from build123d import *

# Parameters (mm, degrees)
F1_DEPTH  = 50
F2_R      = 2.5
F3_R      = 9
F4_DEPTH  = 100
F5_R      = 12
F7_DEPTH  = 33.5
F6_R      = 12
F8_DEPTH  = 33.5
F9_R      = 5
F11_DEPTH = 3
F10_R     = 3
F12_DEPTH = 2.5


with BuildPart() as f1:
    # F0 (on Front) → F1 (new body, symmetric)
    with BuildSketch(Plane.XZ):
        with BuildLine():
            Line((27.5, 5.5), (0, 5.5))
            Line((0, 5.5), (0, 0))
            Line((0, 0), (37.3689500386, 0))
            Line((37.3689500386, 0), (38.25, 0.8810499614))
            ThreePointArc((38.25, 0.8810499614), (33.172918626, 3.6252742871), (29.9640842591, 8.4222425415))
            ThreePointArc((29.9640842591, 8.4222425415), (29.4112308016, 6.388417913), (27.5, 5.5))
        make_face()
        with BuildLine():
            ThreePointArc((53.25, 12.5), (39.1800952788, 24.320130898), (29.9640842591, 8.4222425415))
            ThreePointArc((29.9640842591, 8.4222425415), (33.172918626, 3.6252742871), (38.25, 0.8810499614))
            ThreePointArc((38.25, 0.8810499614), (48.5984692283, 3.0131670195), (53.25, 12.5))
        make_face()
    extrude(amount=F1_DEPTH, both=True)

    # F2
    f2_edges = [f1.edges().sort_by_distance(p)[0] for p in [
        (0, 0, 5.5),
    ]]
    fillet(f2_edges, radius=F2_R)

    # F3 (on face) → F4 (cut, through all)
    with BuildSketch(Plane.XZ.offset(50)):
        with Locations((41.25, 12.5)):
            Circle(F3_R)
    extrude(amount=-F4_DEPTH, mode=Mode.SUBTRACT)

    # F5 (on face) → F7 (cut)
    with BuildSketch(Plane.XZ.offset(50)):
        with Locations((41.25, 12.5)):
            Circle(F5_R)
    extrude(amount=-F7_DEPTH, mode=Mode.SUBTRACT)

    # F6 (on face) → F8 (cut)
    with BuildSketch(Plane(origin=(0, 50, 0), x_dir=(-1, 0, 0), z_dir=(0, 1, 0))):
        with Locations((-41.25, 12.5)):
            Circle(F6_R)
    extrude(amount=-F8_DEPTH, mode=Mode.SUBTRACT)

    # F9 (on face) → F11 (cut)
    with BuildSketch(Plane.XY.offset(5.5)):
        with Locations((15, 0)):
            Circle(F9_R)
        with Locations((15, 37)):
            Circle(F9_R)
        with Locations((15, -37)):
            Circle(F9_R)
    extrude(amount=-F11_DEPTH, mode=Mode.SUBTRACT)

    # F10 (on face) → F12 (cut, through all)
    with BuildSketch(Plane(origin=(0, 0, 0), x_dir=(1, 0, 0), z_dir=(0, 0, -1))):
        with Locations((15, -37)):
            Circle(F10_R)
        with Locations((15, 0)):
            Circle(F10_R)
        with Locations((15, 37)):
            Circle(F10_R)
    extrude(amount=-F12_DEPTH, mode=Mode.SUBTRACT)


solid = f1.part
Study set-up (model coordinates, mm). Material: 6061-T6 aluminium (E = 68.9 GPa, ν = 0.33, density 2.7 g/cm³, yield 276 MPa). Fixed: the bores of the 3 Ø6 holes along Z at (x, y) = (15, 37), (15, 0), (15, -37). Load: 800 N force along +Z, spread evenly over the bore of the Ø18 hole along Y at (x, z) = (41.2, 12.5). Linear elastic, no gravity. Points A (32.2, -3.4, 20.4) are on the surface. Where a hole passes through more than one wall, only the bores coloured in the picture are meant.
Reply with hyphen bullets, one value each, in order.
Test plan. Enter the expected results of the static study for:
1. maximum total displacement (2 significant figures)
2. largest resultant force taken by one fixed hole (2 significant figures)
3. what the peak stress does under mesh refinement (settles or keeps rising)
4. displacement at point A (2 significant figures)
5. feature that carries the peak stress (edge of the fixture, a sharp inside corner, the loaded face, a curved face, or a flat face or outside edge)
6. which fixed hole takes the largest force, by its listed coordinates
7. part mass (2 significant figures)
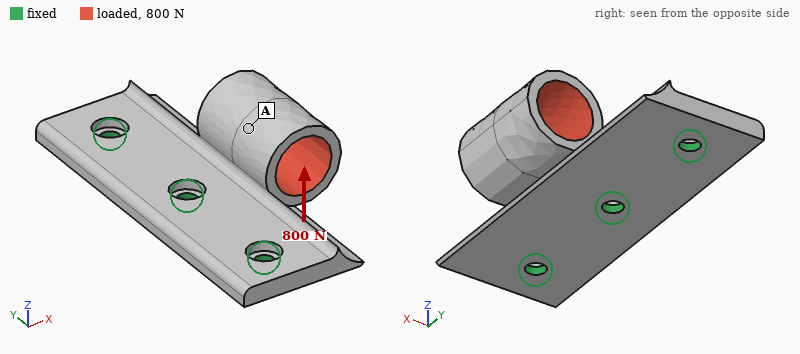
- 0.30 mm
- 580 N
- keeps rising
- 0.18 mm
- edge of the fixture
- (15, 0)
- 67 g
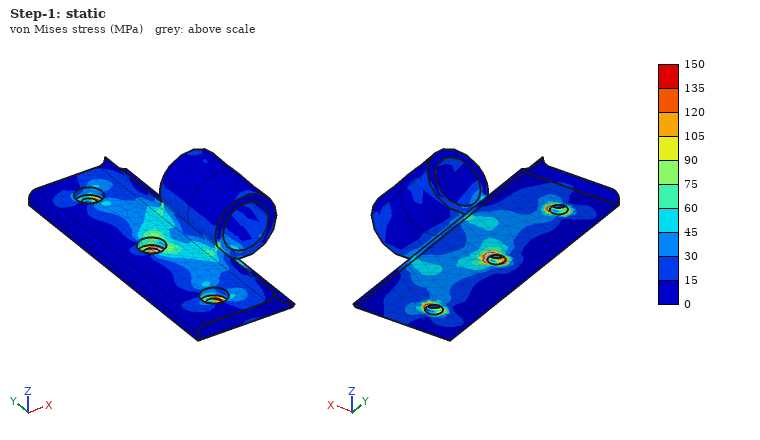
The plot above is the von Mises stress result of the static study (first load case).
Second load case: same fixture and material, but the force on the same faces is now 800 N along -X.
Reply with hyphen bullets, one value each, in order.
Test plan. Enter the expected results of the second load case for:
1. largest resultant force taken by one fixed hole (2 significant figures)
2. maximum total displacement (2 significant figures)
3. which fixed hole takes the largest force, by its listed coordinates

- 510 N
- 0.17 mm
- (15, 0)
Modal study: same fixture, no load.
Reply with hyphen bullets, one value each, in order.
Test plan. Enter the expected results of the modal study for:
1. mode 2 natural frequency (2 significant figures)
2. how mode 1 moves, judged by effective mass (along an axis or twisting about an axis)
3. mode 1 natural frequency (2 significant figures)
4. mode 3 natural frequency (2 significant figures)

- 5700 Hz
- along Z
- 2000 Hz
- 7000 Hz
